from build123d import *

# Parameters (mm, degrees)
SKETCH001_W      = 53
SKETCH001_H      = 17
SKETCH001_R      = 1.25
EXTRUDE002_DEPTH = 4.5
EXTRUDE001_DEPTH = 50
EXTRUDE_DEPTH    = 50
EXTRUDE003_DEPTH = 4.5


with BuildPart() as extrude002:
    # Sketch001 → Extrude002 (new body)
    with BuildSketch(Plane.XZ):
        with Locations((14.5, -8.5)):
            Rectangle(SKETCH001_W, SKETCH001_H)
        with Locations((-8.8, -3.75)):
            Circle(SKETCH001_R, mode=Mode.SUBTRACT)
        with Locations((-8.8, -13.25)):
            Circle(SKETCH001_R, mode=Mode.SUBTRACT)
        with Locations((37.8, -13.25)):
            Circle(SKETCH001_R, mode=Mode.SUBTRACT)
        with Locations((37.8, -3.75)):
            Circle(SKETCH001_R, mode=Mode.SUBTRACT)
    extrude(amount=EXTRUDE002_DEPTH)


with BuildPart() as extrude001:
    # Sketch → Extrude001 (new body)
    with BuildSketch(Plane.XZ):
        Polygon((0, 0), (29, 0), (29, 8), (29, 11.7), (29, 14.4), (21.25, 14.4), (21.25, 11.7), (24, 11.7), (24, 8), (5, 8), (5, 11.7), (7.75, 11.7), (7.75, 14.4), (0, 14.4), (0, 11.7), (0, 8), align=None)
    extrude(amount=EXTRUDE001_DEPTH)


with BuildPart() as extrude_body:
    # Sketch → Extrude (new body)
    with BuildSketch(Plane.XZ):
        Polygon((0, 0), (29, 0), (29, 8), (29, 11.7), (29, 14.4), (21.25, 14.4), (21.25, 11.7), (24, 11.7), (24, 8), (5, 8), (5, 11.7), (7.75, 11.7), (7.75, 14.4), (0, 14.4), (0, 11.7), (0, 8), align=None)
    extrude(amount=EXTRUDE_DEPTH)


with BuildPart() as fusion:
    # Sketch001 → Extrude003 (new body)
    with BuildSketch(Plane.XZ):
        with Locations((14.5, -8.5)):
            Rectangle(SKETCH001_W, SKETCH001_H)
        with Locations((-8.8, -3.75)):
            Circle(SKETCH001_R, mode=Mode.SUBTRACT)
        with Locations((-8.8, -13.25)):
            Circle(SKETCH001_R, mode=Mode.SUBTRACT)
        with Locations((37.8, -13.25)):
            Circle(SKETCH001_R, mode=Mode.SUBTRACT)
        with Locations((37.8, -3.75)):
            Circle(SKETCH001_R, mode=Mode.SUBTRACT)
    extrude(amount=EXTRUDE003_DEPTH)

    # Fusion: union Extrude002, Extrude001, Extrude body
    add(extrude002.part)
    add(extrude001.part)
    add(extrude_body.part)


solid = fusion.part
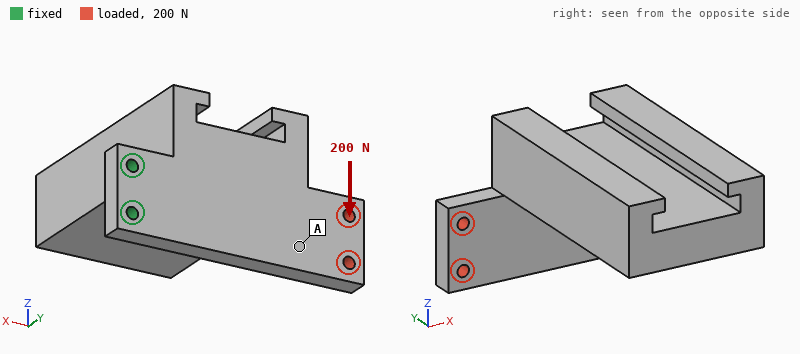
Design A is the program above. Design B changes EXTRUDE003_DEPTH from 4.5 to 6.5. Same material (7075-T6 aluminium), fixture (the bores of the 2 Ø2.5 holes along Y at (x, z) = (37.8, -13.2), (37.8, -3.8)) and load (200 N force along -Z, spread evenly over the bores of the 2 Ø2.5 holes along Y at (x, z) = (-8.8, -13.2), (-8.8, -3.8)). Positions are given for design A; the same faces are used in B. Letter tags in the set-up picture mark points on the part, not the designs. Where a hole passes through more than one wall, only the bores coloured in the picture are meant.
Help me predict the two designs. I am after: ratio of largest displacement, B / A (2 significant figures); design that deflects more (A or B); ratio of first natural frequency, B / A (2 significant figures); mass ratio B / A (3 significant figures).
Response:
0.69
A
1.7
1.09
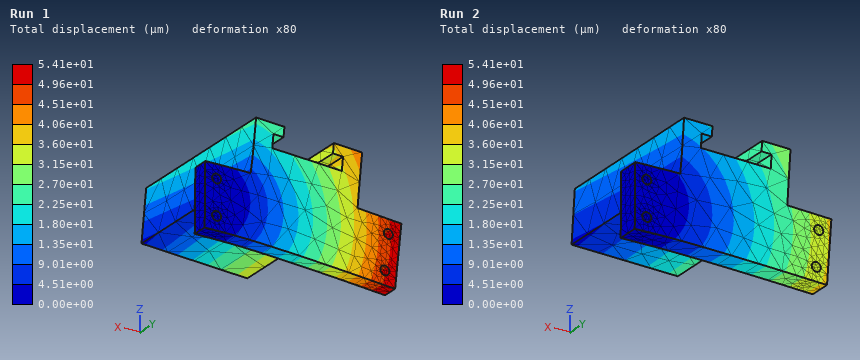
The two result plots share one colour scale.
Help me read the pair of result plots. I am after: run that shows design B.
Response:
Run 2
